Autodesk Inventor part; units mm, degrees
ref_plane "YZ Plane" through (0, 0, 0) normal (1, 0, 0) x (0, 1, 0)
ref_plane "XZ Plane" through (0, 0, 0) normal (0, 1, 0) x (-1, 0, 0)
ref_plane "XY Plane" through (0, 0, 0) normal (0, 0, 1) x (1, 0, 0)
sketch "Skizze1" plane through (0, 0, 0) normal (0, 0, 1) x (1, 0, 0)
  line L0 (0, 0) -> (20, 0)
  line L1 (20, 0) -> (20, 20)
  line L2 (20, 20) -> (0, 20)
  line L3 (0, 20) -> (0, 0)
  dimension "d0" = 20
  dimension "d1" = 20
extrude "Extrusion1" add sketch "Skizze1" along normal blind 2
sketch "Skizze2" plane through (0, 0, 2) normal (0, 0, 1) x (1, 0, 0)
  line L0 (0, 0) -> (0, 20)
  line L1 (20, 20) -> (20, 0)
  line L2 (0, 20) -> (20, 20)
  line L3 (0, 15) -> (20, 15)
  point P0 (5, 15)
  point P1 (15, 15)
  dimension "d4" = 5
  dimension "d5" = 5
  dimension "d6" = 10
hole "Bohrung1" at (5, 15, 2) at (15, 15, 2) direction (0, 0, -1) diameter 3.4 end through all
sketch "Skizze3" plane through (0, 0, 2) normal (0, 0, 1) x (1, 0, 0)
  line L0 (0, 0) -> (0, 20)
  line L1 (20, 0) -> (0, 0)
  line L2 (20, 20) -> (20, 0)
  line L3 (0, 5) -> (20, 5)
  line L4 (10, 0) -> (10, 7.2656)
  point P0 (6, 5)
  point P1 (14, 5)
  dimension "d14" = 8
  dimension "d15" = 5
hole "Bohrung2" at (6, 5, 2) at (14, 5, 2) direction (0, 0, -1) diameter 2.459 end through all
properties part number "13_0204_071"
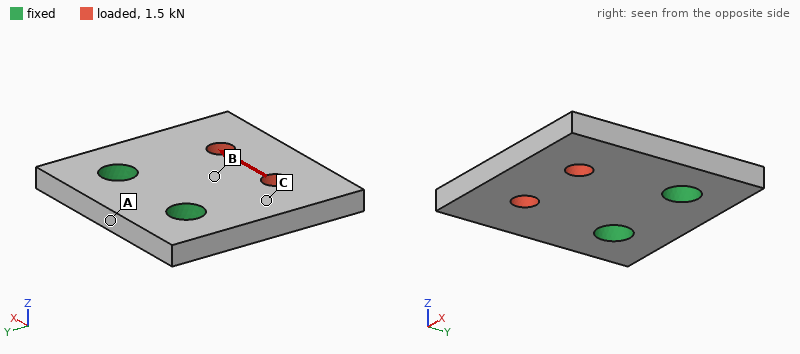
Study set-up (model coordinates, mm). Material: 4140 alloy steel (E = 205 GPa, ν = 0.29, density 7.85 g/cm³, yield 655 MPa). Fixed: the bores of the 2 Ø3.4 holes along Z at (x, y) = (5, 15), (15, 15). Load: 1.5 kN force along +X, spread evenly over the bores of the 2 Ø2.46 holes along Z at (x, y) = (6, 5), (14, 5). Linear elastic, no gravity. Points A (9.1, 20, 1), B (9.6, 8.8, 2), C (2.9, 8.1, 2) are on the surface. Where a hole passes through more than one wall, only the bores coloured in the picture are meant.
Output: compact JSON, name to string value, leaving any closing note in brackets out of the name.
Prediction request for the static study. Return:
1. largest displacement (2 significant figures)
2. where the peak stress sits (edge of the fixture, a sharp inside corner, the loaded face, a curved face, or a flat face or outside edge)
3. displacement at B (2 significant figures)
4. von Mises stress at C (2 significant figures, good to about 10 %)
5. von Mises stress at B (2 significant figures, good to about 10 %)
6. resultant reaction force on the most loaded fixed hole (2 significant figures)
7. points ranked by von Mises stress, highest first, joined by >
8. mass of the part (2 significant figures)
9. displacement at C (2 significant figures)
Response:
{"largest displacement": "11 µm", "where the peak stress sits": "edge of the fixture", "displacement at B": "4.2 µm", "von Mises stress at C": "51 MPa", "von Mises stress at B": "97 MPa", "resultant reaction force on the most loaded fixed hole": "1.3 kN", "points ranked by von Mises stress, highest first, joined by >": "B > C > A", "mass of the part": "5.8 g", "displacement at C": "5.5 µm"}
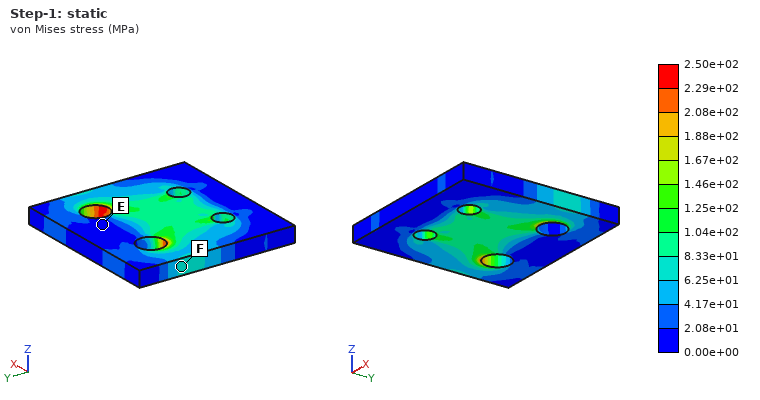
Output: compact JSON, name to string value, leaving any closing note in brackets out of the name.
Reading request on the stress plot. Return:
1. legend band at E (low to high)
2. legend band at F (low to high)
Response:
{"legend band at E": "0.00e+00 to 2.08e+01 MPa", "legend band at F": "6.25e+01 to 8.33e+01 MPa"}
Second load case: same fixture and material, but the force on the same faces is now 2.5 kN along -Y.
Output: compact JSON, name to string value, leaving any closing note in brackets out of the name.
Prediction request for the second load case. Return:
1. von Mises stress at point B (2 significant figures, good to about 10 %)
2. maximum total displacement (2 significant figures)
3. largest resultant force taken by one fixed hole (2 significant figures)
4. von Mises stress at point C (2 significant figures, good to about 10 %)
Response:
{"von Mises stress at point B": "67 MPa", "maximum total displacement": "4.7 µm", "largest resultant force taken by one fixed hole": "1.3 kN", "von Mises stress at point C": "58 MPa"}
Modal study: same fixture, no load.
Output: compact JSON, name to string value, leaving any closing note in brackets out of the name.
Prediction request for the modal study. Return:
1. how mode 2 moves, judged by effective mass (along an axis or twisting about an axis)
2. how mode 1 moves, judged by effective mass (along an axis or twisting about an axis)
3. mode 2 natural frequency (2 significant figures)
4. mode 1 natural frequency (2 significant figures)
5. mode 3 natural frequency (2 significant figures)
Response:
{"how mode 2 moves, judged by effective mass": "twisting about Y", "how mode 1 moves, judged by effective mass": "along Z", "mode 2 natural frequency": "15 kHz", "mode 1 natural frequency": "8400 Hz", "mode 3 natural frequency": "32 kHz"}
